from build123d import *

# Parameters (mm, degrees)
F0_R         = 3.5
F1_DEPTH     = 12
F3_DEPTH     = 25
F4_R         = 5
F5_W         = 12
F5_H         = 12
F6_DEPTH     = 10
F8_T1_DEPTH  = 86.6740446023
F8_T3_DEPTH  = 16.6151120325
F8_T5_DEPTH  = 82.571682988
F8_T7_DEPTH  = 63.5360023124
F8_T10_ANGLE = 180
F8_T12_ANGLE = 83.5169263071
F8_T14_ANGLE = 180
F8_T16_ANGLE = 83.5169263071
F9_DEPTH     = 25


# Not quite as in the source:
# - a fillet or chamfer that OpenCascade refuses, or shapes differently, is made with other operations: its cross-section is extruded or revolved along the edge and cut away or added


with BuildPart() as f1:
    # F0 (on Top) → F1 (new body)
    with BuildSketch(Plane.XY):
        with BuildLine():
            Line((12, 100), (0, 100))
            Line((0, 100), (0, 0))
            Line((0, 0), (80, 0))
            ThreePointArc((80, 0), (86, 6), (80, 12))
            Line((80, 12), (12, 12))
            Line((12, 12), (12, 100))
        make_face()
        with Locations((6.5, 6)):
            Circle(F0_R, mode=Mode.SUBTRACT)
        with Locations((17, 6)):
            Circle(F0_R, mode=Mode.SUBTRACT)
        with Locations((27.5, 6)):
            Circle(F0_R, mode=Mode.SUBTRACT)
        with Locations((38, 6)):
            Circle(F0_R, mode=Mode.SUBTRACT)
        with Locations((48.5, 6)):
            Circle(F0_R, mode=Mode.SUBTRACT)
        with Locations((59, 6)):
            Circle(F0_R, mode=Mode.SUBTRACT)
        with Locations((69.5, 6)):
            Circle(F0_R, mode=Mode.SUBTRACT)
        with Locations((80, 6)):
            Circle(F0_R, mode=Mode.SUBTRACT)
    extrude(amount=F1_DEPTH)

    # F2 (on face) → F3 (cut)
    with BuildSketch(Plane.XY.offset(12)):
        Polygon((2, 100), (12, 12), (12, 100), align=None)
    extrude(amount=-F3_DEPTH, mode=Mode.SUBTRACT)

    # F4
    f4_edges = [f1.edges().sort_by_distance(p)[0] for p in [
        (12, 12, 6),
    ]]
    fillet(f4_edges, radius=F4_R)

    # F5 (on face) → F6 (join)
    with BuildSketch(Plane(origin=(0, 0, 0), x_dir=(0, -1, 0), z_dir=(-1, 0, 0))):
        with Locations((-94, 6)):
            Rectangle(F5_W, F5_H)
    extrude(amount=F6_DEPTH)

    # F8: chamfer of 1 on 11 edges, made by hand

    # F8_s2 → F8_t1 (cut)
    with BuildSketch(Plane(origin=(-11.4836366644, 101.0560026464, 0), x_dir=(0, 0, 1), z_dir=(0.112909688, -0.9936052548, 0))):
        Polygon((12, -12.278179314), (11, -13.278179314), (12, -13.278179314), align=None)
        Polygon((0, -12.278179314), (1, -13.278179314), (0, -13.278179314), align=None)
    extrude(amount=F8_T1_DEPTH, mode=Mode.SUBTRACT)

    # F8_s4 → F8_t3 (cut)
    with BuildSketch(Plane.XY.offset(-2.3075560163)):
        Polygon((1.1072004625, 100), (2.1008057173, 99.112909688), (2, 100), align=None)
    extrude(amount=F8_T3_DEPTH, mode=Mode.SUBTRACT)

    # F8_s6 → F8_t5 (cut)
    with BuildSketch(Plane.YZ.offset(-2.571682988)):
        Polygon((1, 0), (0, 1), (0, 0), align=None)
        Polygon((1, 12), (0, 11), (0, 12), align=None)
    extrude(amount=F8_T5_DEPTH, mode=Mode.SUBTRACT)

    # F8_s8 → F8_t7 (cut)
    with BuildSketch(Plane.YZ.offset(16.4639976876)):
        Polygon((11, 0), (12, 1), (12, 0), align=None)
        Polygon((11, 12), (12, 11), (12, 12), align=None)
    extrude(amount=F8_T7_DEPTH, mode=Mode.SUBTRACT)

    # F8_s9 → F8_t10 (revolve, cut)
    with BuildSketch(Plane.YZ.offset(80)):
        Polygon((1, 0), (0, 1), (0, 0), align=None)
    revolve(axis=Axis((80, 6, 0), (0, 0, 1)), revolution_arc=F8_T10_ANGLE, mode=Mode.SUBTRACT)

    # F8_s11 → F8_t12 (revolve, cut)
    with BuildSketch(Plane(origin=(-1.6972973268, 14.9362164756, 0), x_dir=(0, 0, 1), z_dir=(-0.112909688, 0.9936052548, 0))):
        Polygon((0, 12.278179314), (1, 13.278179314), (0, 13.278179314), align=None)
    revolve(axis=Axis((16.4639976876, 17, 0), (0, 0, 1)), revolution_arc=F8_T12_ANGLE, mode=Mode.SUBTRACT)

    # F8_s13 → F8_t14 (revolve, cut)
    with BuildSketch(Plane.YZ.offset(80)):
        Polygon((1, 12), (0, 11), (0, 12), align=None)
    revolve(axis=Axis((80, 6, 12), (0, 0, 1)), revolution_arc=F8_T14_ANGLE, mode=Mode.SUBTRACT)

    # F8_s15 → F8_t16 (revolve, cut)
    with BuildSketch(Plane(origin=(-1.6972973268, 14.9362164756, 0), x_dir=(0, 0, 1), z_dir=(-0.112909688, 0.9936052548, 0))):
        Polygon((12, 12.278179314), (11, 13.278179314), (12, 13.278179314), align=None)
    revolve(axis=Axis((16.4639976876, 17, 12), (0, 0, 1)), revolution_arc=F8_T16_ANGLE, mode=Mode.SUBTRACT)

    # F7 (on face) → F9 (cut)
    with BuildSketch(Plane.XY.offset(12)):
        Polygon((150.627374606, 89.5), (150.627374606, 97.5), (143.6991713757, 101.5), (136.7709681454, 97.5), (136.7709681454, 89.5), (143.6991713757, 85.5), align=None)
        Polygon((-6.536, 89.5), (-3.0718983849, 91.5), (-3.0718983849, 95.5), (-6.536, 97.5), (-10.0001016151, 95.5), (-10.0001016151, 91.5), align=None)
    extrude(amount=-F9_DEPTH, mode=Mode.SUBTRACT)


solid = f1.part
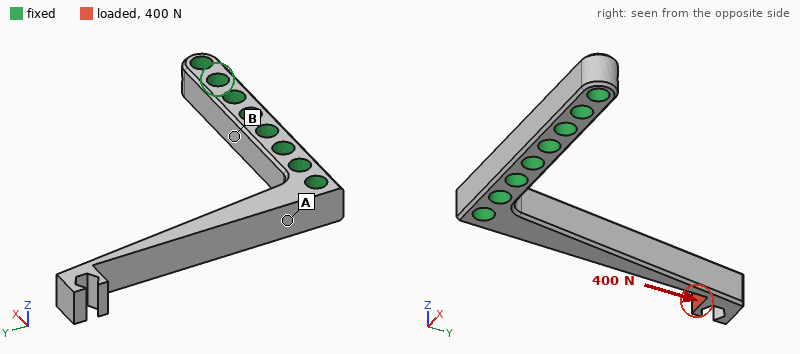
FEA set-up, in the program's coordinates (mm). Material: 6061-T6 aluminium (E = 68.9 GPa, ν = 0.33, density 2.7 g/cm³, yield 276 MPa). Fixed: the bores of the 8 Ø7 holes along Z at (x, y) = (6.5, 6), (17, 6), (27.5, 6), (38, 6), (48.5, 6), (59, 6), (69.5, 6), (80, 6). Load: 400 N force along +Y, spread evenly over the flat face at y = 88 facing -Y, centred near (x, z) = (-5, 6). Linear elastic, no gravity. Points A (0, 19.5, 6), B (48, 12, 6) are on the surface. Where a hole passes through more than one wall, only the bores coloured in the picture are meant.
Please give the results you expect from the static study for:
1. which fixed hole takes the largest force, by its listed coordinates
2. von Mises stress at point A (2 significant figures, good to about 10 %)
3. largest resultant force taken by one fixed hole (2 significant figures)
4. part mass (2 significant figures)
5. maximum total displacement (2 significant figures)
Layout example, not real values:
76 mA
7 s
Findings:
(6.5, 6)
20 MPa
650 N
45 g
0.58 mm
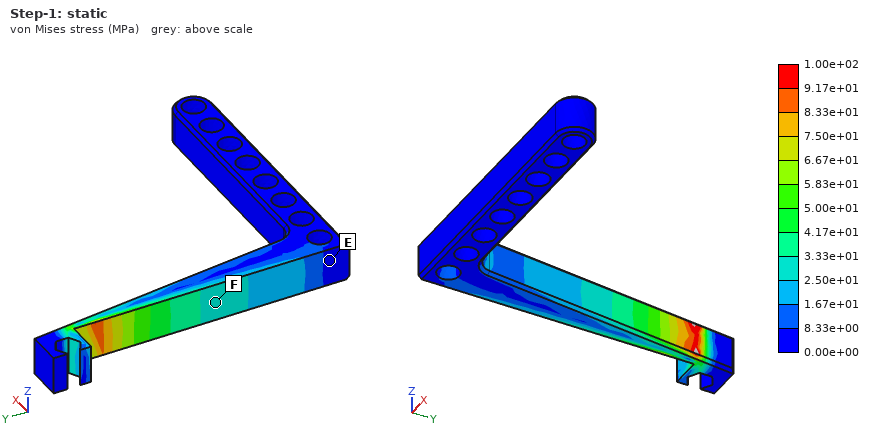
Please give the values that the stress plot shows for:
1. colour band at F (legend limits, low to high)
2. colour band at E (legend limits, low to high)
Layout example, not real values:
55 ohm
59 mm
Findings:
2.50e+01 to 3.33e+01 MPa
0.00e+00 to 8.33e+00 MPa
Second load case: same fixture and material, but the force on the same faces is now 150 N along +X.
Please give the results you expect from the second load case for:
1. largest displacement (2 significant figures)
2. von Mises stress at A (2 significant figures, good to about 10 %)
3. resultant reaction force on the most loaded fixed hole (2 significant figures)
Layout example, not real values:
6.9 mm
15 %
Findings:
0.66 mm
42 MPa
890 N
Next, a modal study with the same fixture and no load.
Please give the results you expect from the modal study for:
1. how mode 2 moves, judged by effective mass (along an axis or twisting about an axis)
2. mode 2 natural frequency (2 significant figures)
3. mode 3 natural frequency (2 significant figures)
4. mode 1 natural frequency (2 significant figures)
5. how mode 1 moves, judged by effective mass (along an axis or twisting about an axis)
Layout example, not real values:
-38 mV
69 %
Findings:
along Z
1400 Hz
3900 Hz
1100 Hz
along X
